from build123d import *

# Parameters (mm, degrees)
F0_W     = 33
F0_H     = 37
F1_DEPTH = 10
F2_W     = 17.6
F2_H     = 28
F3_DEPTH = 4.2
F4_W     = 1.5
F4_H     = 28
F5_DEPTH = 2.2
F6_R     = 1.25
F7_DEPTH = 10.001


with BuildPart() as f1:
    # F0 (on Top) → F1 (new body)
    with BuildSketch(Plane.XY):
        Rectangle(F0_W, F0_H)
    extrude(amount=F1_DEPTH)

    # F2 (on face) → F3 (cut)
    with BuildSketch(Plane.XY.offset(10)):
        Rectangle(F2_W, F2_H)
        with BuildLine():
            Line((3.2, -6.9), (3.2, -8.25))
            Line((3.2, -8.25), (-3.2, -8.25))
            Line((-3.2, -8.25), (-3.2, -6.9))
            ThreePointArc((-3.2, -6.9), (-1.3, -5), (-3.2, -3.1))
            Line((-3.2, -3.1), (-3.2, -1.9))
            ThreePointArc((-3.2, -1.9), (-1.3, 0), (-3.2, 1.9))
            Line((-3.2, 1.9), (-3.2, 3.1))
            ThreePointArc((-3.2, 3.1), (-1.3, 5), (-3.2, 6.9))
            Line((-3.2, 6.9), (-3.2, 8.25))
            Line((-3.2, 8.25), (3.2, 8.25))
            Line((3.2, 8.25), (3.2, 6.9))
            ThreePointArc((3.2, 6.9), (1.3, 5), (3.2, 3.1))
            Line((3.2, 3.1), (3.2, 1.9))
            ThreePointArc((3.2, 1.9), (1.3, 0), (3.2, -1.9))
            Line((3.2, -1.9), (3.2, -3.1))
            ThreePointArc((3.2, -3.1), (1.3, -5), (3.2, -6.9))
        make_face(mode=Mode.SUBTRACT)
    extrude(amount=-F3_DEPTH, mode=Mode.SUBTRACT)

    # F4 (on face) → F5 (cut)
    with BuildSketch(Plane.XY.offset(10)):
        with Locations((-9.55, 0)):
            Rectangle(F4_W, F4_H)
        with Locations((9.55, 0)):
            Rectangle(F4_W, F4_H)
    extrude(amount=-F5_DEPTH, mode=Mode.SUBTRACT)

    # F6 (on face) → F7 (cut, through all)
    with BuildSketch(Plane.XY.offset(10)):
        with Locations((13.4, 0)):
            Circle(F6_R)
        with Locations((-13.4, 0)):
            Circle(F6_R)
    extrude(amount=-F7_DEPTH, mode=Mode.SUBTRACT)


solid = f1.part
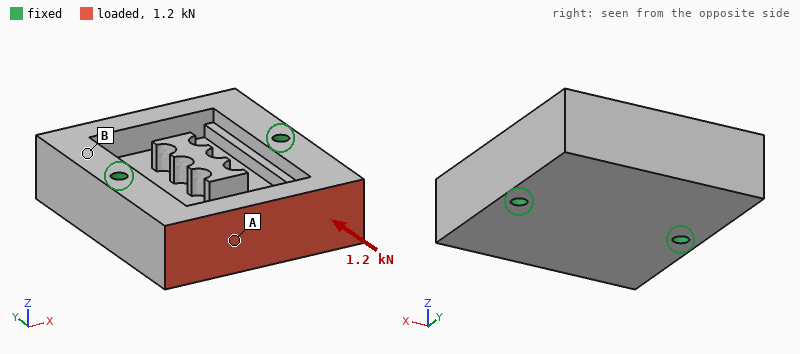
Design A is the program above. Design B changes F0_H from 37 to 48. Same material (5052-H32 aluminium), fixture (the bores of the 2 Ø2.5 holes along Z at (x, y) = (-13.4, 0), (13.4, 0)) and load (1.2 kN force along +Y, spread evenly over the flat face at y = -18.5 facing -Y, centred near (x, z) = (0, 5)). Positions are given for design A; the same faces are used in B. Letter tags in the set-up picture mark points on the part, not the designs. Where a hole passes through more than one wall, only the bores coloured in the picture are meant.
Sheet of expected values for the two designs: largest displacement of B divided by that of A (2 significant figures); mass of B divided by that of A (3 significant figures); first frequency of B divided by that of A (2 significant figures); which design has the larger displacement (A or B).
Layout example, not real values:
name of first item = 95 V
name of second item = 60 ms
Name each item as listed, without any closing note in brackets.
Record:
largest displacement of B divided by that of A = 0.80
mass of B divided by that of A = 1.36
first frequency of B divided by that of A = 0.64
which design has the larger displacement = A
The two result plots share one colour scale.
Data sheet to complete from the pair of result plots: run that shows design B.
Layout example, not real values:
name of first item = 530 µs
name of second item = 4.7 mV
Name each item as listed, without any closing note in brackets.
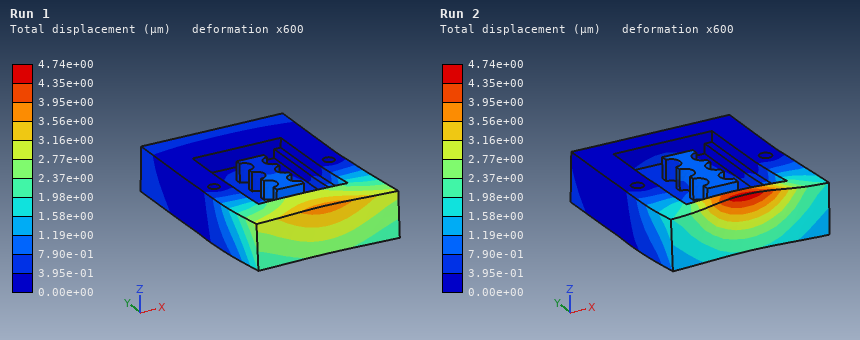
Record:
run that shows design B = Run 1
